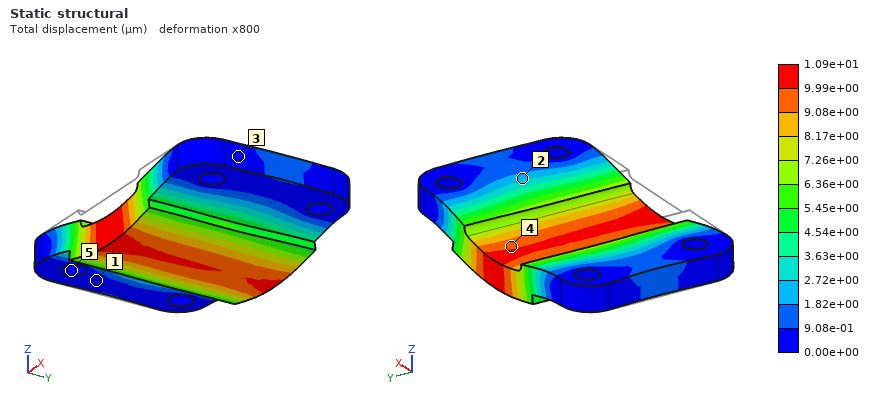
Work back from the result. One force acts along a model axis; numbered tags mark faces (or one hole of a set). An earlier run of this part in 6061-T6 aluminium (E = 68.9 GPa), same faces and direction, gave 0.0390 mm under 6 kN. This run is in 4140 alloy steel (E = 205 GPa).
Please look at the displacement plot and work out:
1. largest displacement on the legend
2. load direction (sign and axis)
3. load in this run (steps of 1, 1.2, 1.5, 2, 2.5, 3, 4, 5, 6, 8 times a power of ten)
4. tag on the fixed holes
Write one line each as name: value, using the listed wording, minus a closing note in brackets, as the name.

largest displacement on the legend: 1.09e+01 µm
load direction: -Z
load in this run: 5 kN
tag on the fixed holes: 5
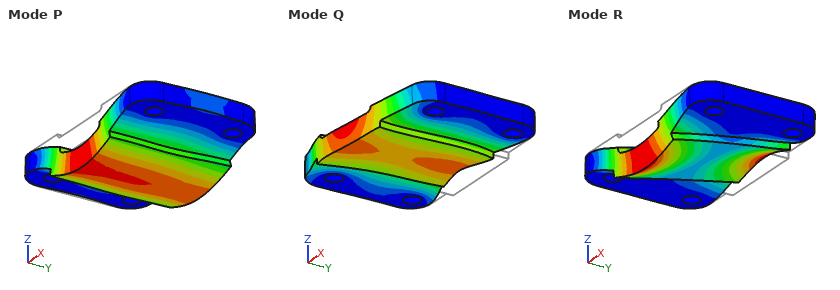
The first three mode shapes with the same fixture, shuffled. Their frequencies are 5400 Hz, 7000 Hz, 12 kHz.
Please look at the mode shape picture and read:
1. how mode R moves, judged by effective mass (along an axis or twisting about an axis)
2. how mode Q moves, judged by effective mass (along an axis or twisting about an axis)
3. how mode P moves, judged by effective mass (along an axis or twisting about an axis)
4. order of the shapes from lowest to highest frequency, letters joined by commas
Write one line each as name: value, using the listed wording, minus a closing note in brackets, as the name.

how mode R moves, judged by effective mass: twisting about X
how mode Q moves, judged by effective mass: along Y
how mode P moves, judged by effective mass: along Z
order of the shapes from lowest to highest frequency, letters joined by commas: P, R, Q
